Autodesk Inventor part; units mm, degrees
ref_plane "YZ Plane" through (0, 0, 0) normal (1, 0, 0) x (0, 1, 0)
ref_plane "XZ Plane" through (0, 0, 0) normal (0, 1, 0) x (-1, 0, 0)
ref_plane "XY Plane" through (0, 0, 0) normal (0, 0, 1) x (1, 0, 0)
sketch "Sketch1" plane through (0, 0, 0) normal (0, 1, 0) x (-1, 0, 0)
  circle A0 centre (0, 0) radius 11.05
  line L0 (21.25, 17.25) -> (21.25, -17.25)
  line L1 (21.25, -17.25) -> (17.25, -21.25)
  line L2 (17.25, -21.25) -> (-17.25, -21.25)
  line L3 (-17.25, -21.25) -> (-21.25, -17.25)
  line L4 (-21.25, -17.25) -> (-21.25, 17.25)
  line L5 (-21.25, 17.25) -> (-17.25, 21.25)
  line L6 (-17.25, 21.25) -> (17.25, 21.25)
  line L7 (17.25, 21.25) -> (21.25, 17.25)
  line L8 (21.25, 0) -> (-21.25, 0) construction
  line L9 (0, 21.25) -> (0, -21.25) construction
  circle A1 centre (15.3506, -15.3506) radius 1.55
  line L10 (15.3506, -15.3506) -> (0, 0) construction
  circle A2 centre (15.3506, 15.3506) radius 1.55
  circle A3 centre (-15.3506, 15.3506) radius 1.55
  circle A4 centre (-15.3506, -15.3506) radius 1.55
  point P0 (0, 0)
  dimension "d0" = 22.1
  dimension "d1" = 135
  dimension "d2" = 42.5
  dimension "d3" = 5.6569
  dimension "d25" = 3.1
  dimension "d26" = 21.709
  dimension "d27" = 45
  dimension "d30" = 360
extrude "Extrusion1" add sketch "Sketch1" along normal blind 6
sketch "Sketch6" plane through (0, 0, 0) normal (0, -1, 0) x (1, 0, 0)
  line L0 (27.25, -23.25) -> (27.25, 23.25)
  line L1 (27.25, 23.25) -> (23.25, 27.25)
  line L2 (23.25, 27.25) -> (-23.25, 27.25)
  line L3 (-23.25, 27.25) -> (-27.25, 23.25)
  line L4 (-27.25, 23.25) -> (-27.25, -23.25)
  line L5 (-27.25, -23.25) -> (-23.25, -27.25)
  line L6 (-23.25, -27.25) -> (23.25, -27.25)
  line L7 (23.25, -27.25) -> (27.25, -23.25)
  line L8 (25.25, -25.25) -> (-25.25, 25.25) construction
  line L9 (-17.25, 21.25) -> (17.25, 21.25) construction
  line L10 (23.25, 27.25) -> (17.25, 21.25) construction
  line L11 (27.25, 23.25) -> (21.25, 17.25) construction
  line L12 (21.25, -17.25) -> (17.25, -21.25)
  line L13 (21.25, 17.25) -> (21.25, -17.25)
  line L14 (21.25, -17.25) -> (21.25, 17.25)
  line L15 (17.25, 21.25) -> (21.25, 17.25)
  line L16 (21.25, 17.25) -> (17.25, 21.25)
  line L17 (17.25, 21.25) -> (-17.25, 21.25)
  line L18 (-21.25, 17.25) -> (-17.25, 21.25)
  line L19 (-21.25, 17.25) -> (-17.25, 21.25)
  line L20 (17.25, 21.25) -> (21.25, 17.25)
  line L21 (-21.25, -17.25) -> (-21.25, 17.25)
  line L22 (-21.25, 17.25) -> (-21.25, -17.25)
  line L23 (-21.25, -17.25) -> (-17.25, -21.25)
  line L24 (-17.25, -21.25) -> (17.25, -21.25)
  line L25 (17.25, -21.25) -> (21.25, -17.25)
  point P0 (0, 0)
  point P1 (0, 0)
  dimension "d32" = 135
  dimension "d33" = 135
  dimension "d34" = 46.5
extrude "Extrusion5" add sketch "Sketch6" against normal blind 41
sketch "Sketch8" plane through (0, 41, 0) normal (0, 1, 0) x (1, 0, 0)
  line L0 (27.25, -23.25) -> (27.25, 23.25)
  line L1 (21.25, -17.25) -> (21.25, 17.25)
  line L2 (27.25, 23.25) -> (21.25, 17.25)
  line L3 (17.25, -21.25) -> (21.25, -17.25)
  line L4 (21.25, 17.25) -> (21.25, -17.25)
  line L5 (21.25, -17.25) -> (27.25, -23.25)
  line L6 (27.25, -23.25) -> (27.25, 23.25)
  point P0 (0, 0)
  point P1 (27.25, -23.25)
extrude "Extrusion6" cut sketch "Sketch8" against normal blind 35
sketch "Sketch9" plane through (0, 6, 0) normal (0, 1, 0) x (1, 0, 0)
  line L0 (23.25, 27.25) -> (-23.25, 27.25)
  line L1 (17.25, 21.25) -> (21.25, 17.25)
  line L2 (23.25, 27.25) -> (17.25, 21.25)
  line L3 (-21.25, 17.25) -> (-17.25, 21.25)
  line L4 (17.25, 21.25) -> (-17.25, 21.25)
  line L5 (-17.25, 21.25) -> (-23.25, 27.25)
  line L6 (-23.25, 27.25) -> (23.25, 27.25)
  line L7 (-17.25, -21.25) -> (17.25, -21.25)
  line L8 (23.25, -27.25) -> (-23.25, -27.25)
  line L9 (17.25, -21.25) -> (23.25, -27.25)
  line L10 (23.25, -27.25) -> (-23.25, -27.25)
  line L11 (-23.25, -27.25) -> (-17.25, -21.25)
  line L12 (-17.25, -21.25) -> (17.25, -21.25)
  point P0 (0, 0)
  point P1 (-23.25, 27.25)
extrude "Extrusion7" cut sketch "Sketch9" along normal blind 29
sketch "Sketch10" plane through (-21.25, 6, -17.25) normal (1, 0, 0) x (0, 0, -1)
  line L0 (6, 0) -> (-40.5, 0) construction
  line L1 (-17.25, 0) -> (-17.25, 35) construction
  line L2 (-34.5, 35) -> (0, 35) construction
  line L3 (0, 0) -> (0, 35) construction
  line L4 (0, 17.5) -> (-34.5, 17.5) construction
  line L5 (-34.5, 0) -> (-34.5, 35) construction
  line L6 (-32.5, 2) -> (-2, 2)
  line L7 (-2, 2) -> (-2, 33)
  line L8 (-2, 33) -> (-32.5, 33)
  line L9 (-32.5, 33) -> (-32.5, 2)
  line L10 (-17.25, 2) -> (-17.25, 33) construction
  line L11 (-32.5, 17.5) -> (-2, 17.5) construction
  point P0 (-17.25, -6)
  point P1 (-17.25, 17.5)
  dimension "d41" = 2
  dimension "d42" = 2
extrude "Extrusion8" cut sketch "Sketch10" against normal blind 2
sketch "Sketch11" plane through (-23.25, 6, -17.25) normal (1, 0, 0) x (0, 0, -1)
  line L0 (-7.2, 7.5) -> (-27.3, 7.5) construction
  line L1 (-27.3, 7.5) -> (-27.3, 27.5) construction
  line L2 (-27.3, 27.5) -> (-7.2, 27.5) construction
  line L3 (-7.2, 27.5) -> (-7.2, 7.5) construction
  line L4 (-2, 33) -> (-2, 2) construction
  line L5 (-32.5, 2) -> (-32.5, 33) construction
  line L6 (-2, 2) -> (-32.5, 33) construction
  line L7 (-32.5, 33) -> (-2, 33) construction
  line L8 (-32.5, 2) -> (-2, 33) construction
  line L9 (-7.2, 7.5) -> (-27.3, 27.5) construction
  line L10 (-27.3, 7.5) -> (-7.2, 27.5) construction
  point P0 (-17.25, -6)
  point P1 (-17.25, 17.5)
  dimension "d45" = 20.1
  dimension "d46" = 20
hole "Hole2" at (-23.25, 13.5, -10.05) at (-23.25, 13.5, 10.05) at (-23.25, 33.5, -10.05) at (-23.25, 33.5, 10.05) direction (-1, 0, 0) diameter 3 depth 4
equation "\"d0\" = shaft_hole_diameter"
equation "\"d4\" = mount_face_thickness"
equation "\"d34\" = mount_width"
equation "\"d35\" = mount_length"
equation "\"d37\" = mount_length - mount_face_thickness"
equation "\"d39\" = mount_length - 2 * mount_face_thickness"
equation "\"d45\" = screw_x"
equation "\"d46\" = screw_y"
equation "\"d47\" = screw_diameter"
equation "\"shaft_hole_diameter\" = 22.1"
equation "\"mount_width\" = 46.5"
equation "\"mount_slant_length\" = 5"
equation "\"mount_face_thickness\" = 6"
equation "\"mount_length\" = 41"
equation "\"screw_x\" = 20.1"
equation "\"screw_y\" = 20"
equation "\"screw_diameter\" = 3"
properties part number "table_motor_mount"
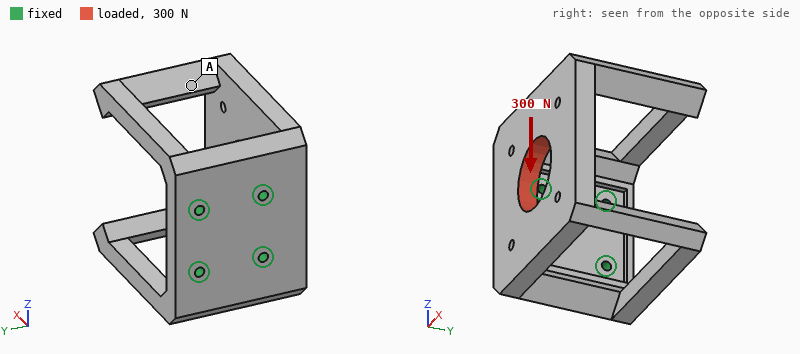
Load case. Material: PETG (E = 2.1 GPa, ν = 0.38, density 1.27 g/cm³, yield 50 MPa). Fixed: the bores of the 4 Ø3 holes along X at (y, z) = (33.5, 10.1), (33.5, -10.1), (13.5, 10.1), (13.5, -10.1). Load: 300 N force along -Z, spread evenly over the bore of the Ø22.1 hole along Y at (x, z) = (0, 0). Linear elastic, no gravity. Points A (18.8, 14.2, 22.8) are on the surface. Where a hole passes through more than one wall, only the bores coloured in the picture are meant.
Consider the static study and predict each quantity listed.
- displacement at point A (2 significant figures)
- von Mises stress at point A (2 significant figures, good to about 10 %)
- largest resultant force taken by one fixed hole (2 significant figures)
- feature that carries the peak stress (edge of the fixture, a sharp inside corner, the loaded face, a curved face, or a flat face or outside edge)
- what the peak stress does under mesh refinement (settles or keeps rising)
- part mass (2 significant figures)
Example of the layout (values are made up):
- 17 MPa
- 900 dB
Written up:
- 0.84 mm
- 2.7 MPa
- 350 N
- edge of the fixture
- keeps rising
- 40 g
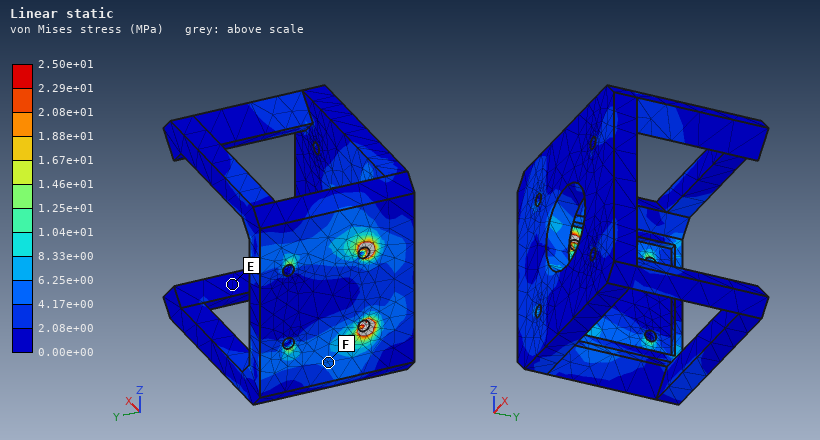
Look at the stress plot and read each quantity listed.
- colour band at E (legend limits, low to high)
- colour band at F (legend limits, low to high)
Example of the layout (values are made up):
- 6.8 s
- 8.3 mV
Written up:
- 0.00e+00 to 2.08e+00 MPa
- 4.17e+00 to 6.25e+00 MPa
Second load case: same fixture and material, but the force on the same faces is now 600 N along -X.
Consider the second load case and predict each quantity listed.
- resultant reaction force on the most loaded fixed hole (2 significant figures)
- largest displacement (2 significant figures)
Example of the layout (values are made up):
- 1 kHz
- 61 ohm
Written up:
- 400 N
- 0.98 mm
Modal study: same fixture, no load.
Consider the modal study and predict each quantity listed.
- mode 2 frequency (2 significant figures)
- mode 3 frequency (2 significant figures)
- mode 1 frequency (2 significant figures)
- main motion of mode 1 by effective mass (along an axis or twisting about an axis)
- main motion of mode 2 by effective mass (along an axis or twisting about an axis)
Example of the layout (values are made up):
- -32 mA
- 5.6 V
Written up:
- 470 Hz
- 750 Hz
- 420 Hz
- along Y
- along Z
